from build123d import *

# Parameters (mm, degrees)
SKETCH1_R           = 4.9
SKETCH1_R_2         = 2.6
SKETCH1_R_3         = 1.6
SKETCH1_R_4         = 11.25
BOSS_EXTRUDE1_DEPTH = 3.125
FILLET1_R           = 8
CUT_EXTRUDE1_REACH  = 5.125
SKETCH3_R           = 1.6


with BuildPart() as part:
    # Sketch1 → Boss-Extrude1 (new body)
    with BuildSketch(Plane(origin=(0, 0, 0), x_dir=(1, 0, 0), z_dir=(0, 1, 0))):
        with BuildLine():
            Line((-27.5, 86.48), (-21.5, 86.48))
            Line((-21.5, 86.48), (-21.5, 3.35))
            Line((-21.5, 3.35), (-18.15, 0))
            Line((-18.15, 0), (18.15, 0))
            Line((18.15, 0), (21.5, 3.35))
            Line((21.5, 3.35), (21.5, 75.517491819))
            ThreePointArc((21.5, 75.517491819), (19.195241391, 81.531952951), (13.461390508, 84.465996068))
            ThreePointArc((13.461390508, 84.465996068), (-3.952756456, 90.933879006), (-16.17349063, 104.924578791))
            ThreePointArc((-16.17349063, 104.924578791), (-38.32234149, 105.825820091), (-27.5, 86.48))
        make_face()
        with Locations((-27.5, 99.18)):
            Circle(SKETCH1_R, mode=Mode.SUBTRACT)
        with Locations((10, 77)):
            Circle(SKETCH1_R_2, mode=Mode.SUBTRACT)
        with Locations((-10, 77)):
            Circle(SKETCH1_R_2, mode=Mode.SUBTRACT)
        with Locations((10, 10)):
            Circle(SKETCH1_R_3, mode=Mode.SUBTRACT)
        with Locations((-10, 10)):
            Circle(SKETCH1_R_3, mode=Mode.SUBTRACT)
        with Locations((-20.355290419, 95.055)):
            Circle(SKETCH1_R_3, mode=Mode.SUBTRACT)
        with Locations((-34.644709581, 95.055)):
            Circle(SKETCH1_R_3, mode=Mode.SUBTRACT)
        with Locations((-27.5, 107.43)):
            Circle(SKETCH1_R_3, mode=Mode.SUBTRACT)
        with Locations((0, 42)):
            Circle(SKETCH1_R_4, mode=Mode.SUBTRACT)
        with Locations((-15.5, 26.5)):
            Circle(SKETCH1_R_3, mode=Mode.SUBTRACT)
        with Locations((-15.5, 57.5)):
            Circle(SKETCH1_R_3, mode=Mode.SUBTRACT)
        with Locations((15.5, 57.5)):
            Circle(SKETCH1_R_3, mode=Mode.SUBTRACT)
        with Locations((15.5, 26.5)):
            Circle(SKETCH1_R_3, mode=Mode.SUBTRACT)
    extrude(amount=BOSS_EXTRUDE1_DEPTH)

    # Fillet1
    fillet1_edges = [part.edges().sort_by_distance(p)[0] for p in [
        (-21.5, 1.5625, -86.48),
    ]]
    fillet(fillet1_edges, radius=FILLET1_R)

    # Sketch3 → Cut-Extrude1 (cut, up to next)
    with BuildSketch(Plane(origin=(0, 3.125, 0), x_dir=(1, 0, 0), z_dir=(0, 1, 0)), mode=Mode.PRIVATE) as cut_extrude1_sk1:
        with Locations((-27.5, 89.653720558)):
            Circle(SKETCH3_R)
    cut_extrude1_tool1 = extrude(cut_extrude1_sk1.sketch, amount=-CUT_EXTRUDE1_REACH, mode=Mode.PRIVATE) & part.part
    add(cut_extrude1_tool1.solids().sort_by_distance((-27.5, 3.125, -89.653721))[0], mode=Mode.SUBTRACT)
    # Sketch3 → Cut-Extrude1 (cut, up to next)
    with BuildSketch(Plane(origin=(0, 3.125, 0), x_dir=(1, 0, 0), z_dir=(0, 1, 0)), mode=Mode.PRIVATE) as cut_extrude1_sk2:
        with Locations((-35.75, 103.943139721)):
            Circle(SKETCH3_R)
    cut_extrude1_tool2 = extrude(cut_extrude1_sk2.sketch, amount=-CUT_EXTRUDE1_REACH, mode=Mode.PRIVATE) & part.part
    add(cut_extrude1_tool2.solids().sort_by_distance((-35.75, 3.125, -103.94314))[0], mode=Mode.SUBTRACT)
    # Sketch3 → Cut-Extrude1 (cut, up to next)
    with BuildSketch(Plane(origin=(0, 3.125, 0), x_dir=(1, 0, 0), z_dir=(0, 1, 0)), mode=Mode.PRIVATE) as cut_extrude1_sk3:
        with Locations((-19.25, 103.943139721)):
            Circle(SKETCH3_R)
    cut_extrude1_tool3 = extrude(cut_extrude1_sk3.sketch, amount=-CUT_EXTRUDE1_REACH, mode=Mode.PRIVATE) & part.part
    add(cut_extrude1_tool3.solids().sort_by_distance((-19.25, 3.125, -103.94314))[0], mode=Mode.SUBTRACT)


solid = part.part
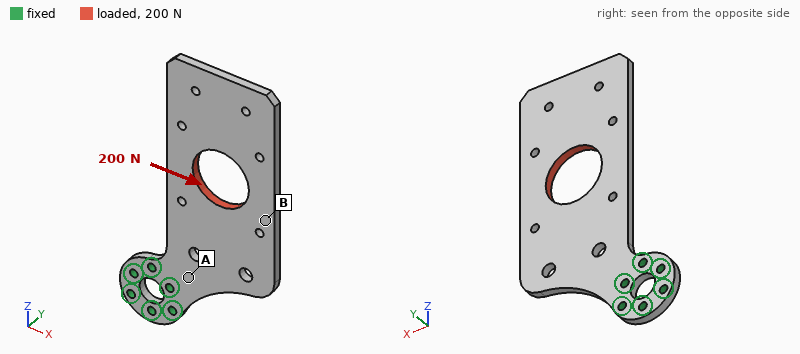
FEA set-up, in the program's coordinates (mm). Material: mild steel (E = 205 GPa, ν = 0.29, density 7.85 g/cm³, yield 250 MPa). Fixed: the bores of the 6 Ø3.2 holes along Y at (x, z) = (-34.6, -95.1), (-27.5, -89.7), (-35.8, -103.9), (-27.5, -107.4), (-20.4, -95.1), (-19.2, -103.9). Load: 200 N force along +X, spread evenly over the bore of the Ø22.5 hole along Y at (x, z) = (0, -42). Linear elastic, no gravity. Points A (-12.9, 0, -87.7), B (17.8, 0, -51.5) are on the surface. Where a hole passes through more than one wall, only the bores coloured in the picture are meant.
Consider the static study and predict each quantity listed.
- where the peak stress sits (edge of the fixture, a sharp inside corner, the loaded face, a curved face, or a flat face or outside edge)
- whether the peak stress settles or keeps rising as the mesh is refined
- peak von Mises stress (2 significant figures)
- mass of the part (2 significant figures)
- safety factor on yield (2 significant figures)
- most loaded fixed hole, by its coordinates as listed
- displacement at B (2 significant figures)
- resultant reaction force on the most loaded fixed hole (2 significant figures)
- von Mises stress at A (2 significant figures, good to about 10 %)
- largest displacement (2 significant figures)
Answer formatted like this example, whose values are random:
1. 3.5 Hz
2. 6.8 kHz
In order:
1. a curved face
2. settles
3. 87 MPa
4. 91 g
5. 2.9
6. (-27.5, -89.7)
7. 29 µm
8. 760 N
9. 15 MPa
10. 55 µm
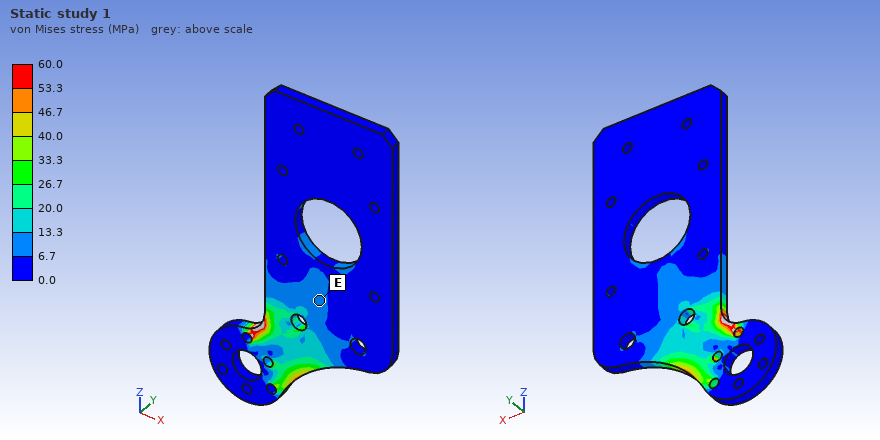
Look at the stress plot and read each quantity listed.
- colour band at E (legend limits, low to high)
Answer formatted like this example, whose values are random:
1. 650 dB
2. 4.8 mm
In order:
1. 6.7 to 13.3 MPa
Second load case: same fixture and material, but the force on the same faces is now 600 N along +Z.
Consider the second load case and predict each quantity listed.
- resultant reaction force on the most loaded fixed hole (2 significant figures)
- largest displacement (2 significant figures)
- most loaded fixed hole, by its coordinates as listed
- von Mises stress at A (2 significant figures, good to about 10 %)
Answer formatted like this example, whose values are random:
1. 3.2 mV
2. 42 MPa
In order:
1. 750 N
2. 57 µm
3. (-27.5, -89.7)
4. 24 MPa
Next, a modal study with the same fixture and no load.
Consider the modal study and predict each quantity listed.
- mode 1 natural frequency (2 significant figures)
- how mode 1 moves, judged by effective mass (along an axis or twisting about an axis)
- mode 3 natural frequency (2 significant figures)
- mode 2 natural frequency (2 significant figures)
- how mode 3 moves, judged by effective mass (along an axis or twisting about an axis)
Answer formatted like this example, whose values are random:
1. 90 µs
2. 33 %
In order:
1. 210 Hz
2. along Y
3. 1300 Hz
4. 810 Hz
5. along X
